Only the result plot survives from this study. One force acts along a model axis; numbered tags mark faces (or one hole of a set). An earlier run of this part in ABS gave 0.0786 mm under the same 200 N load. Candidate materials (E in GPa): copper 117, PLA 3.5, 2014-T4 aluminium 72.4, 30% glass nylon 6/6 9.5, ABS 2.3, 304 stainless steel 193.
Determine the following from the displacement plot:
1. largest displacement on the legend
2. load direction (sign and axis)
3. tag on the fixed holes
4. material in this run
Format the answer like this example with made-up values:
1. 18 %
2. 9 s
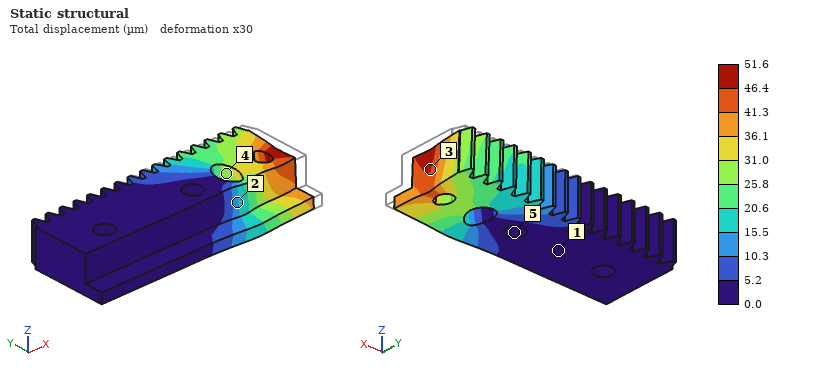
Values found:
1. 51.6 µm
2. -X
3. 5
4. PLA
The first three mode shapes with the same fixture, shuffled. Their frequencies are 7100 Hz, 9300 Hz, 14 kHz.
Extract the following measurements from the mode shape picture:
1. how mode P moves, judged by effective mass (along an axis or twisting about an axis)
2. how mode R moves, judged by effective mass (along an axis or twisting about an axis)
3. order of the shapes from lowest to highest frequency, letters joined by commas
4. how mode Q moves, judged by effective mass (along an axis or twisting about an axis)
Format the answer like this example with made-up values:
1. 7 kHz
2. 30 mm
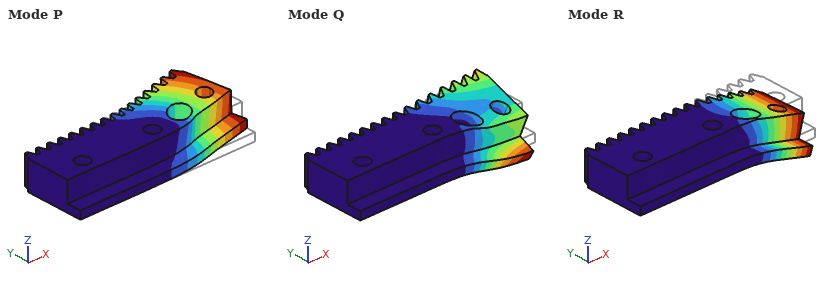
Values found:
1. along Y
2. along Z
3. R, P, Q
4. twisting about X
